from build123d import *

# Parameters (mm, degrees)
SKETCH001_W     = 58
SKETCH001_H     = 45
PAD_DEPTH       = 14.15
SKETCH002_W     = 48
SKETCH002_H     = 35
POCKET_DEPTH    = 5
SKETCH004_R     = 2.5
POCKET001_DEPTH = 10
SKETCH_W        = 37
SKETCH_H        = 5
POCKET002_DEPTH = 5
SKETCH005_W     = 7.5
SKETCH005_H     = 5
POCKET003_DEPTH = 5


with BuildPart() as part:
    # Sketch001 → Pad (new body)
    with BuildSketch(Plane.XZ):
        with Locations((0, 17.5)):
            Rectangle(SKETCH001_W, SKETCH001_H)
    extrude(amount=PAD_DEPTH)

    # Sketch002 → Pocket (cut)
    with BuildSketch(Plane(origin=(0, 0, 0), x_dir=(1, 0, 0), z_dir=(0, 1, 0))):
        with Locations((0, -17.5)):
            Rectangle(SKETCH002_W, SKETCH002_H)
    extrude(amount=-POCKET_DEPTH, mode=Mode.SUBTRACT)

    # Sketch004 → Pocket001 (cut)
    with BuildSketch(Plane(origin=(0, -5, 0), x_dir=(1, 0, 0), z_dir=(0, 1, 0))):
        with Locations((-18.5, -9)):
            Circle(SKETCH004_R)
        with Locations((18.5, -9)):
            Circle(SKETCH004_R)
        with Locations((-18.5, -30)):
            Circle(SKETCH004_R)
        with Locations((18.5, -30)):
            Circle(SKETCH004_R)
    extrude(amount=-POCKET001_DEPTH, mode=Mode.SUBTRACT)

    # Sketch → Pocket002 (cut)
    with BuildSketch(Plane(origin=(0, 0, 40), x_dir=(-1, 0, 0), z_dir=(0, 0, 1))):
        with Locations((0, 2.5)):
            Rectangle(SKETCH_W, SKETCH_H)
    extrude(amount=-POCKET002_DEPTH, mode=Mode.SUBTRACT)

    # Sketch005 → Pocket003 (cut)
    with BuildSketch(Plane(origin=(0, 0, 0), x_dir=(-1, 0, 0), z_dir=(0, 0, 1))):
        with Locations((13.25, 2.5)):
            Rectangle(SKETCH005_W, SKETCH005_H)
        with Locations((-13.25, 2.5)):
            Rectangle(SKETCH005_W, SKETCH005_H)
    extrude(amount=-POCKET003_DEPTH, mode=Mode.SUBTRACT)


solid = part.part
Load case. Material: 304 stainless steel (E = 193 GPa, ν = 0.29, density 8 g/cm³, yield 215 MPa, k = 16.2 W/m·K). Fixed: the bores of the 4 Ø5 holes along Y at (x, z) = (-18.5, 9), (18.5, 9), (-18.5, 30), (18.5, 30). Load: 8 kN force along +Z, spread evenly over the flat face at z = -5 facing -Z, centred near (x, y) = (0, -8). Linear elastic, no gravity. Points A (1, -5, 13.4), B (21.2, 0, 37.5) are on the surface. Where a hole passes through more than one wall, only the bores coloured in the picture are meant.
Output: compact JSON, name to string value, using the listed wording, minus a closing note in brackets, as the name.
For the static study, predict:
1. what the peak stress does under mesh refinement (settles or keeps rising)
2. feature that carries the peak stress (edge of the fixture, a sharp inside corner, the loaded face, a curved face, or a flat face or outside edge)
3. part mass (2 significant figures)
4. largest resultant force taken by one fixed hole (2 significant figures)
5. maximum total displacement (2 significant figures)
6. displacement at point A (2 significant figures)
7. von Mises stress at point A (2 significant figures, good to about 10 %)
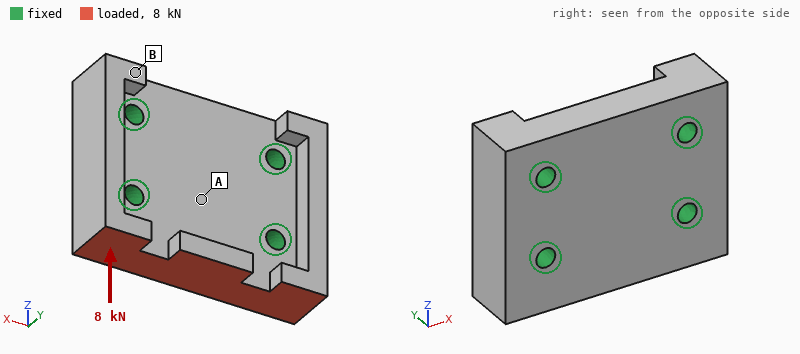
{"what the peak stress does under mesh refinement": "keeps rising", "feature that carries the peak stress": "edge of the fixture", "part mass": "210 g", "largest resultant force taken by one fixed hole": "3.0 kN", "maximum total displacement": "7.1 µm", "displacement at point A": "1.2 µm", "von Mises stress at point A": "15 MPa"}
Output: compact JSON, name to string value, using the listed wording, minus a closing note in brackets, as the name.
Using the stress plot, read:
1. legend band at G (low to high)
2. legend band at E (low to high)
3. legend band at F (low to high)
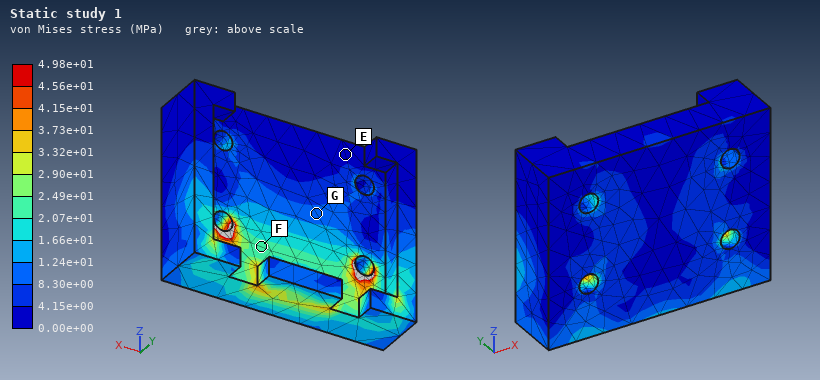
{"legend band at G": "8.30e+00 to 1.24e+01 MPa", "legend band at E": "0.00e+00 to 4.15e+00 MPa", "legend band at F": "2.07e+01 to 2.49e+01 MPa"}
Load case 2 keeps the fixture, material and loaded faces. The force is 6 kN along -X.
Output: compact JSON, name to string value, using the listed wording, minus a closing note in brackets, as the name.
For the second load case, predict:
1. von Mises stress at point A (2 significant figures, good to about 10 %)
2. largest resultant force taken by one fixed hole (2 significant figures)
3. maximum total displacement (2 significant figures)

{"von Mises stress at point A": "8.1 MPa", "largest resultant force taken by one fixed hole": "3.3 kN", "maximum total displacement": "5.7 µm"}
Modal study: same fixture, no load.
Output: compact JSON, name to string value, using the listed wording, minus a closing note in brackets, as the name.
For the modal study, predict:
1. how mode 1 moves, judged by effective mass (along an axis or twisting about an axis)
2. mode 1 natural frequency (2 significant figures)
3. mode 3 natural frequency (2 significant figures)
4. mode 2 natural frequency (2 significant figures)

{"how mode 1 moves, judged by effective mass": "along Y", "mode 1 natural frequency": "19 kHz", "mode 3 natural frequency": "26 kHz", "mode 2 natural frequency": "24 kHz"}
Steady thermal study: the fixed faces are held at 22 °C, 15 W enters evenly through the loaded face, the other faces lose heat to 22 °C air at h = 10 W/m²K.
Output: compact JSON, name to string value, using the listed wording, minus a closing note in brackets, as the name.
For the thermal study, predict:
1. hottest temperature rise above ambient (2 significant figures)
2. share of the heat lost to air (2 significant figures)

{"hottest temperature rise above ambient": "33 K", "share of the heat lost to air": "3.5 %"}
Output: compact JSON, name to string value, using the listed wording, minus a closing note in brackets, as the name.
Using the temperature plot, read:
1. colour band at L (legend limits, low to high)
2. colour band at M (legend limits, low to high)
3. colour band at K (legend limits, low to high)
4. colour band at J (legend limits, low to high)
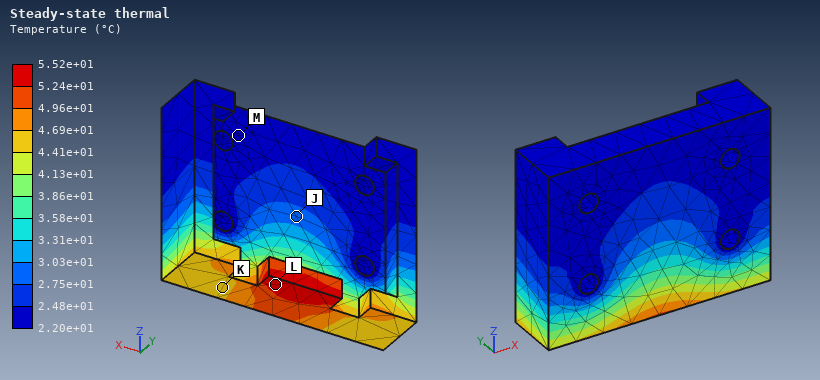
{"colour band at L": "5.24e+01 to 5.52e+01 °C", "colour band at M": "2.20e+01 to 2.48e+01 °C", "colour band at K": "4.41e+01 to 4.69e+01 °C", "colour band at J": "2.75e+01 to 3.03e+01 °C"}
